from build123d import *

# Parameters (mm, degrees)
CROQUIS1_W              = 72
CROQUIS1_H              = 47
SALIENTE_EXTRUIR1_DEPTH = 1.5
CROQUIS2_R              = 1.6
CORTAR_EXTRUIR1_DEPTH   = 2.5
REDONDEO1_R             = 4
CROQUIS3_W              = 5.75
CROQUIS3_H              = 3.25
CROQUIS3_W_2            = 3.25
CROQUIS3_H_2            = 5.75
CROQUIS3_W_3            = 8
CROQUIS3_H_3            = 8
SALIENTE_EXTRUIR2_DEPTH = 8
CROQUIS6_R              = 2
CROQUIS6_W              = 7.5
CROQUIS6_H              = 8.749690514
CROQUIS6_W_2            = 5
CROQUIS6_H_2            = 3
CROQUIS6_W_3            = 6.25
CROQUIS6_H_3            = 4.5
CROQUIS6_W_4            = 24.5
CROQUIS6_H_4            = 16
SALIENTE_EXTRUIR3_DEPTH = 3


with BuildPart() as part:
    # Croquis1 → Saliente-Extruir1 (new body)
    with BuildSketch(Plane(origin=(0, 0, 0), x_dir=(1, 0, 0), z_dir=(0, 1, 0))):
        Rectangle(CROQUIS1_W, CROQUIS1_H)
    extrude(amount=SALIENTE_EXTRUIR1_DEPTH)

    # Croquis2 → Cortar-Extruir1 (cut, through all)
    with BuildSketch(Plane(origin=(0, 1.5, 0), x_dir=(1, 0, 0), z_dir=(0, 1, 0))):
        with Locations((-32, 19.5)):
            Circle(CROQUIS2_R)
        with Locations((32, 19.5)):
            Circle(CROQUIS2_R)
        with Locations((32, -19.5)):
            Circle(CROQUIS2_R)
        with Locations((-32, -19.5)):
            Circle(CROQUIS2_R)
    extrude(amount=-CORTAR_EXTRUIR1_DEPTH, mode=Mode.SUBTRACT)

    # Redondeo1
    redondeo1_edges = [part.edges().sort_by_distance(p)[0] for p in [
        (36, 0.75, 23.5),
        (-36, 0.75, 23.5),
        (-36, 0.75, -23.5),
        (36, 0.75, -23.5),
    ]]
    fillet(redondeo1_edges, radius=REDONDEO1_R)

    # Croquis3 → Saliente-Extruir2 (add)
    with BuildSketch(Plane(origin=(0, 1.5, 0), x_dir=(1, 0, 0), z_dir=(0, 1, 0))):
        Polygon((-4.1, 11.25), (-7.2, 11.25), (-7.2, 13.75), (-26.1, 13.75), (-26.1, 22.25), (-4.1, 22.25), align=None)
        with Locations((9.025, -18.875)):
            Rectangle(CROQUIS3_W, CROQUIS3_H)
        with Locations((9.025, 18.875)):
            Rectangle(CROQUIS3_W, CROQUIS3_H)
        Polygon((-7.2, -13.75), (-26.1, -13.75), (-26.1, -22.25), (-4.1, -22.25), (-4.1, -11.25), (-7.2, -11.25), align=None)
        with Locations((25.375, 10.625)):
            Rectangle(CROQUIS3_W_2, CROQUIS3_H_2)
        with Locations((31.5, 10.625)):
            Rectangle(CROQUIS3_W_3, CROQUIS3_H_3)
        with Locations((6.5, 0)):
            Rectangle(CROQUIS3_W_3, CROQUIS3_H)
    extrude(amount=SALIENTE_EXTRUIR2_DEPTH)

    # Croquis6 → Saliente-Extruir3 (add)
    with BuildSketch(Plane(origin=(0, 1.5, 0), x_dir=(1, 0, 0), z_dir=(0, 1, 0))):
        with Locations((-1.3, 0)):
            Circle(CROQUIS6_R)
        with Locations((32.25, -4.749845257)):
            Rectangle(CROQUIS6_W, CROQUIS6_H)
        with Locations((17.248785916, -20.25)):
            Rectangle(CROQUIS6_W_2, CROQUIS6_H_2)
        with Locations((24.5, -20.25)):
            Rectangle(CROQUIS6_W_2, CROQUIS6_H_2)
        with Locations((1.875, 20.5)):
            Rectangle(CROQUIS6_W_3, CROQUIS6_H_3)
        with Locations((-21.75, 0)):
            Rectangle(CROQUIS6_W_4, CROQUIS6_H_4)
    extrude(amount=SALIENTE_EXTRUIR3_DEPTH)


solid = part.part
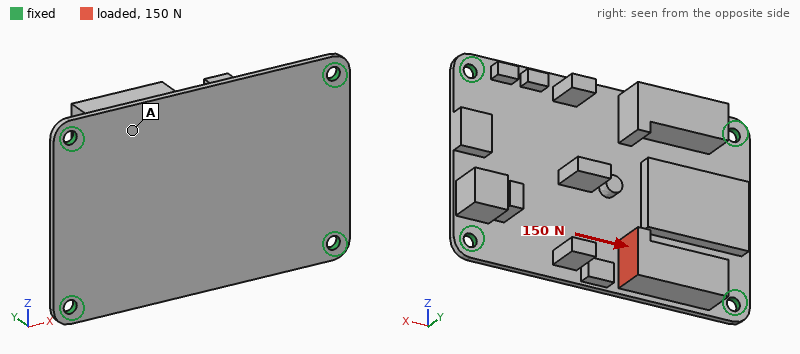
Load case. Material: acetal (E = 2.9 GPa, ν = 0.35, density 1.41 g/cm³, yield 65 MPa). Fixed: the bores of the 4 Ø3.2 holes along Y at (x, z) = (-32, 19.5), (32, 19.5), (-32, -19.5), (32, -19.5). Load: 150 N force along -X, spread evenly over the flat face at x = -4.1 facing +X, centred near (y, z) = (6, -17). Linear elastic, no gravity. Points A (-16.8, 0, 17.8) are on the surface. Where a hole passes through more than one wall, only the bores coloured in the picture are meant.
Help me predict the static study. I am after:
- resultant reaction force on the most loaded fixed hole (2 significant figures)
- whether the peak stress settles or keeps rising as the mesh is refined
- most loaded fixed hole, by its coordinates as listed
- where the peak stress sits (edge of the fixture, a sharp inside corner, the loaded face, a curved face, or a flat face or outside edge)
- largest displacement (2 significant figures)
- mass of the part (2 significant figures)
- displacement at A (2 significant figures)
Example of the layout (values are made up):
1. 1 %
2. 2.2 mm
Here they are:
1. 76 N
2. keeps rising
3. (-32, -19.5)
4. edge of the fixture
5. 1.0 mm
6. 15 g
7. 0.24 mm
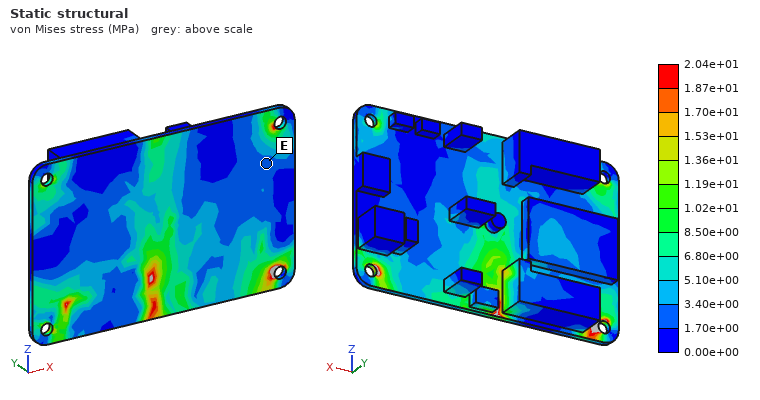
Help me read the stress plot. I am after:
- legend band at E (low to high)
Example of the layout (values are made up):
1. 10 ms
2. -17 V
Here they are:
1. 1.70e+00 to 3.40e+00 MPa
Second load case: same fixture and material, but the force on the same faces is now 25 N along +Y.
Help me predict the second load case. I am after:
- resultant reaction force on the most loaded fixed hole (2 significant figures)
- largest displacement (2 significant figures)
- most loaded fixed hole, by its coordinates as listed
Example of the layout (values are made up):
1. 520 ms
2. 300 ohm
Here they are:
1. 19 N
2. 0.89 mm
3. (-32, -19.5)
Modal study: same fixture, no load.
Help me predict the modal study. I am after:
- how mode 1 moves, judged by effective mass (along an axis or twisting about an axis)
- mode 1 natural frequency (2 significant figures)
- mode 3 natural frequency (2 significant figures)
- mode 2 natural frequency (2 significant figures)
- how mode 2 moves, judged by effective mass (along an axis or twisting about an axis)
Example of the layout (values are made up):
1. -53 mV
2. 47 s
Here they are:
1. along Y
2. 410 Hz
3. 1100 Hz
4. 820 Hz
5. twisting about X
